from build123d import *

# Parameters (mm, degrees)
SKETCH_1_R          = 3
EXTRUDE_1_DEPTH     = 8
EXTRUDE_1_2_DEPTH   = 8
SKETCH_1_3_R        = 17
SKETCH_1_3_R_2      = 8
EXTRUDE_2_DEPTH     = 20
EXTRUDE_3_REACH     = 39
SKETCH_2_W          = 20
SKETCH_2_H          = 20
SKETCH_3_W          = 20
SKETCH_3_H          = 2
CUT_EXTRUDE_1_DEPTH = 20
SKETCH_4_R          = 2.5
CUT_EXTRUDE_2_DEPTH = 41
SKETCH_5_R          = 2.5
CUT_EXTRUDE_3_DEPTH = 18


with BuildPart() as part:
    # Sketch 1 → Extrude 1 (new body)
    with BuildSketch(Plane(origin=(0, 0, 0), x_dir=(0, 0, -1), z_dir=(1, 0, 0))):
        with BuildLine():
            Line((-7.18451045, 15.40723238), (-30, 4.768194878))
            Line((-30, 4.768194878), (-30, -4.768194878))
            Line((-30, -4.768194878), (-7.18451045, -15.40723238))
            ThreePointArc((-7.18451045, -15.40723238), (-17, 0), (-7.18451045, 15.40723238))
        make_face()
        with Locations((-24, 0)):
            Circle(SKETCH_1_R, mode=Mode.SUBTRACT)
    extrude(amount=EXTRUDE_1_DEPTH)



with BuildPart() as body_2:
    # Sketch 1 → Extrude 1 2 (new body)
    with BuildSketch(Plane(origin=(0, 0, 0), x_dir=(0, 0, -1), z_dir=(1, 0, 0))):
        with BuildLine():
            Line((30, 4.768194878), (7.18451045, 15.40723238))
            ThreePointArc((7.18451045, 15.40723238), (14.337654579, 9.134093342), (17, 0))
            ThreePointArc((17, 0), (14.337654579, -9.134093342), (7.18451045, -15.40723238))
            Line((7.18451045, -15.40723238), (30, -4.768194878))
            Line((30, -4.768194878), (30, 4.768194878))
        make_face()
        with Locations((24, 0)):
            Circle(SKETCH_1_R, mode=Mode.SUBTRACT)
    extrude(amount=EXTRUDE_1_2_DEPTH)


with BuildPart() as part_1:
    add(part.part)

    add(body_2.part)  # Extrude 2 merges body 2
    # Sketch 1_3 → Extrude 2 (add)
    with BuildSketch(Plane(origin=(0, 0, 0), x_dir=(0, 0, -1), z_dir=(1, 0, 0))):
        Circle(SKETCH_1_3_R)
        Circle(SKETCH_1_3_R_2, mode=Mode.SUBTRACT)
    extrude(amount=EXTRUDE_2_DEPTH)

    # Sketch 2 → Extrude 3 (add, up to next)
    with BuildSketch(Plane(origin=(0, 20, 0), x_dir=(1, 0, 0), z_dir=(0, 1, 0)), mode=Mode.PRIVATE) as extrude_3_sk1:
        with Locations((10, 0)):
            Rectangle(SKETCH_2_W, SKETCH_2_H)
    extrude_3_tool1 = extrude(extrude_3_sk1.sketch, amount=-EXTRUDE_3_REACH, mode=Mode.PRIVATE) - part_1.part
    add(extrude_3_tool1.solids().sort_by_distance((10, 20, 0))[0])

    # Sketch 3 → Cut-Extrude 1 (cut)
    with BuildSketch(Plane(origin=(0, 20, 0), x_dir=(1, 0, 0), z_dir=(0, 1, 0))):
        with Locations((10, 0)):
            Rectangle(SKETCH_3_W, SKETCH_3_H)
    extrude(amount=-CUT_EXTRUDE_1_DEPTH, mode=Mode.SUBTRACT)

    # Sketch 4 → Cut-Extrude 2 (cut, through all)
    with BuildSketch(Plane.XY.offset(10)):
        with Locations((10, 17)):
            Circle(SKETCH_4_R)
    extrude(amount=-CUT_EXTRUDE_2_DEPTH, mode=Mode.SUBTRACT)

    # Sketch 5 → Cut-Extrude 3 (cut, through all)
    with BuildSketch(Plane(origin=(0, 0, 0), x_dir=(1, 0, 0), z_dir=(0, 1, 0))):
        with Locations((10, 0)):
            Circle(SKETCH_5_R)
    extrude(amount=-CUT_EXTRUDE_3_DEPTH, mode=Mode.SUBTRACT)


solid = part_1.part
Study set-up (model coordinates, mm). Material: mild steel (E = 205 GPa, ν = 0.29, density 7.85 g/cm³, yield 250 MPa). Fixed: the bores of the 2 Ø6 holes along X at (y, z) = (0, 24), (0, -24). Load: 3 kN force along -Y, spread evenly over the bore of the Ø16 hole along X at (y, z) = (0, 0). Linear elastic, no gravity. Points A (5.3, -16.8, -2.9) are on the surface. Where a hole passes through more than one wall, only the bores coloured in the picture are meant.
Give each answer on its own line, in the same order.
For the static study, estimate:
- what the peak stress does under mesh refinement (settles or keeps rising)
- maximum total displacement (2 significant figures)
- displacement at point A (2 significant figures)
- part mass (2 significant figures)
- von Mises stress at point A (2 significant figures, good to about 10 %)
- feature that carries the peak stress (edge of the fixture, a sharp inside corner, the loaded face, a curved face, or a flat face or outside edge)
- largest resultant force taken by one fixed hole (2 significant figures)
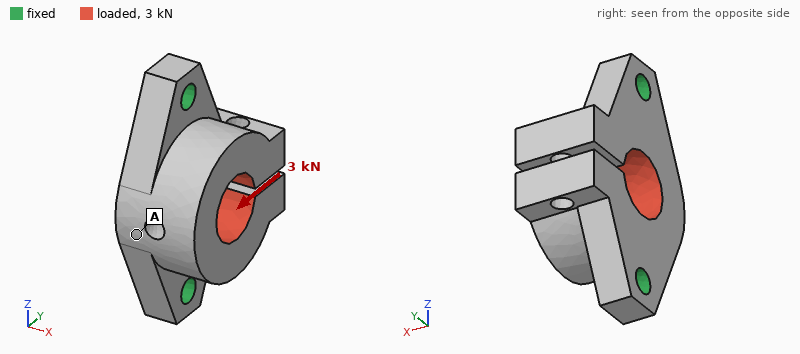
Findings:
keeps rising
15 µm
8.3 µm
140 g
14 MPa
edge of the fixture
2.0 kN
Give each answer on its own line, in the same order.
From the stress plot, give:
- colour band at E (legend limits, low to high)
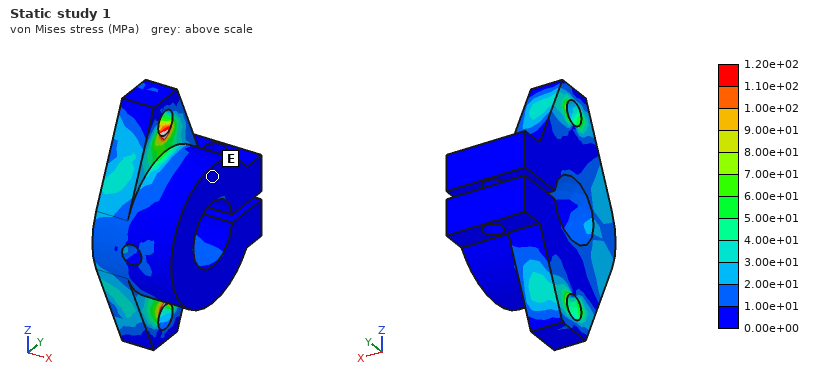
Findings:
0.00e+00 to 1.00e+01 MPa
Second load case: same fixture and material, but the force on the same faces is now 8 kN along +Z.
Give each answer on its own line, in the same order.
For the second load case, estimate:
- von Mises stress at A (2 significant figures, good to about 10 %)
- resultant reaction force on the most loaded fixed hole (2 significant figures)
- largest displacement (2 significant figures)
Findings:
12 MPa
4.1 kN
17 µm
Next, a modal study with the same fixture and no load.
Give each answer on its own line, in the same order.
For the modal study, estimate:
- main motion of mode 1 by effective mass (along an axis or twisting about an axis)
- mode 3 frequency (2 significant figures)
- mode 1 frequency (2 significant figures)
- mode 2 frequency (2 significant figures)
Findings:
along Y
9000 Hz
7200 Hz
8400 Hz
